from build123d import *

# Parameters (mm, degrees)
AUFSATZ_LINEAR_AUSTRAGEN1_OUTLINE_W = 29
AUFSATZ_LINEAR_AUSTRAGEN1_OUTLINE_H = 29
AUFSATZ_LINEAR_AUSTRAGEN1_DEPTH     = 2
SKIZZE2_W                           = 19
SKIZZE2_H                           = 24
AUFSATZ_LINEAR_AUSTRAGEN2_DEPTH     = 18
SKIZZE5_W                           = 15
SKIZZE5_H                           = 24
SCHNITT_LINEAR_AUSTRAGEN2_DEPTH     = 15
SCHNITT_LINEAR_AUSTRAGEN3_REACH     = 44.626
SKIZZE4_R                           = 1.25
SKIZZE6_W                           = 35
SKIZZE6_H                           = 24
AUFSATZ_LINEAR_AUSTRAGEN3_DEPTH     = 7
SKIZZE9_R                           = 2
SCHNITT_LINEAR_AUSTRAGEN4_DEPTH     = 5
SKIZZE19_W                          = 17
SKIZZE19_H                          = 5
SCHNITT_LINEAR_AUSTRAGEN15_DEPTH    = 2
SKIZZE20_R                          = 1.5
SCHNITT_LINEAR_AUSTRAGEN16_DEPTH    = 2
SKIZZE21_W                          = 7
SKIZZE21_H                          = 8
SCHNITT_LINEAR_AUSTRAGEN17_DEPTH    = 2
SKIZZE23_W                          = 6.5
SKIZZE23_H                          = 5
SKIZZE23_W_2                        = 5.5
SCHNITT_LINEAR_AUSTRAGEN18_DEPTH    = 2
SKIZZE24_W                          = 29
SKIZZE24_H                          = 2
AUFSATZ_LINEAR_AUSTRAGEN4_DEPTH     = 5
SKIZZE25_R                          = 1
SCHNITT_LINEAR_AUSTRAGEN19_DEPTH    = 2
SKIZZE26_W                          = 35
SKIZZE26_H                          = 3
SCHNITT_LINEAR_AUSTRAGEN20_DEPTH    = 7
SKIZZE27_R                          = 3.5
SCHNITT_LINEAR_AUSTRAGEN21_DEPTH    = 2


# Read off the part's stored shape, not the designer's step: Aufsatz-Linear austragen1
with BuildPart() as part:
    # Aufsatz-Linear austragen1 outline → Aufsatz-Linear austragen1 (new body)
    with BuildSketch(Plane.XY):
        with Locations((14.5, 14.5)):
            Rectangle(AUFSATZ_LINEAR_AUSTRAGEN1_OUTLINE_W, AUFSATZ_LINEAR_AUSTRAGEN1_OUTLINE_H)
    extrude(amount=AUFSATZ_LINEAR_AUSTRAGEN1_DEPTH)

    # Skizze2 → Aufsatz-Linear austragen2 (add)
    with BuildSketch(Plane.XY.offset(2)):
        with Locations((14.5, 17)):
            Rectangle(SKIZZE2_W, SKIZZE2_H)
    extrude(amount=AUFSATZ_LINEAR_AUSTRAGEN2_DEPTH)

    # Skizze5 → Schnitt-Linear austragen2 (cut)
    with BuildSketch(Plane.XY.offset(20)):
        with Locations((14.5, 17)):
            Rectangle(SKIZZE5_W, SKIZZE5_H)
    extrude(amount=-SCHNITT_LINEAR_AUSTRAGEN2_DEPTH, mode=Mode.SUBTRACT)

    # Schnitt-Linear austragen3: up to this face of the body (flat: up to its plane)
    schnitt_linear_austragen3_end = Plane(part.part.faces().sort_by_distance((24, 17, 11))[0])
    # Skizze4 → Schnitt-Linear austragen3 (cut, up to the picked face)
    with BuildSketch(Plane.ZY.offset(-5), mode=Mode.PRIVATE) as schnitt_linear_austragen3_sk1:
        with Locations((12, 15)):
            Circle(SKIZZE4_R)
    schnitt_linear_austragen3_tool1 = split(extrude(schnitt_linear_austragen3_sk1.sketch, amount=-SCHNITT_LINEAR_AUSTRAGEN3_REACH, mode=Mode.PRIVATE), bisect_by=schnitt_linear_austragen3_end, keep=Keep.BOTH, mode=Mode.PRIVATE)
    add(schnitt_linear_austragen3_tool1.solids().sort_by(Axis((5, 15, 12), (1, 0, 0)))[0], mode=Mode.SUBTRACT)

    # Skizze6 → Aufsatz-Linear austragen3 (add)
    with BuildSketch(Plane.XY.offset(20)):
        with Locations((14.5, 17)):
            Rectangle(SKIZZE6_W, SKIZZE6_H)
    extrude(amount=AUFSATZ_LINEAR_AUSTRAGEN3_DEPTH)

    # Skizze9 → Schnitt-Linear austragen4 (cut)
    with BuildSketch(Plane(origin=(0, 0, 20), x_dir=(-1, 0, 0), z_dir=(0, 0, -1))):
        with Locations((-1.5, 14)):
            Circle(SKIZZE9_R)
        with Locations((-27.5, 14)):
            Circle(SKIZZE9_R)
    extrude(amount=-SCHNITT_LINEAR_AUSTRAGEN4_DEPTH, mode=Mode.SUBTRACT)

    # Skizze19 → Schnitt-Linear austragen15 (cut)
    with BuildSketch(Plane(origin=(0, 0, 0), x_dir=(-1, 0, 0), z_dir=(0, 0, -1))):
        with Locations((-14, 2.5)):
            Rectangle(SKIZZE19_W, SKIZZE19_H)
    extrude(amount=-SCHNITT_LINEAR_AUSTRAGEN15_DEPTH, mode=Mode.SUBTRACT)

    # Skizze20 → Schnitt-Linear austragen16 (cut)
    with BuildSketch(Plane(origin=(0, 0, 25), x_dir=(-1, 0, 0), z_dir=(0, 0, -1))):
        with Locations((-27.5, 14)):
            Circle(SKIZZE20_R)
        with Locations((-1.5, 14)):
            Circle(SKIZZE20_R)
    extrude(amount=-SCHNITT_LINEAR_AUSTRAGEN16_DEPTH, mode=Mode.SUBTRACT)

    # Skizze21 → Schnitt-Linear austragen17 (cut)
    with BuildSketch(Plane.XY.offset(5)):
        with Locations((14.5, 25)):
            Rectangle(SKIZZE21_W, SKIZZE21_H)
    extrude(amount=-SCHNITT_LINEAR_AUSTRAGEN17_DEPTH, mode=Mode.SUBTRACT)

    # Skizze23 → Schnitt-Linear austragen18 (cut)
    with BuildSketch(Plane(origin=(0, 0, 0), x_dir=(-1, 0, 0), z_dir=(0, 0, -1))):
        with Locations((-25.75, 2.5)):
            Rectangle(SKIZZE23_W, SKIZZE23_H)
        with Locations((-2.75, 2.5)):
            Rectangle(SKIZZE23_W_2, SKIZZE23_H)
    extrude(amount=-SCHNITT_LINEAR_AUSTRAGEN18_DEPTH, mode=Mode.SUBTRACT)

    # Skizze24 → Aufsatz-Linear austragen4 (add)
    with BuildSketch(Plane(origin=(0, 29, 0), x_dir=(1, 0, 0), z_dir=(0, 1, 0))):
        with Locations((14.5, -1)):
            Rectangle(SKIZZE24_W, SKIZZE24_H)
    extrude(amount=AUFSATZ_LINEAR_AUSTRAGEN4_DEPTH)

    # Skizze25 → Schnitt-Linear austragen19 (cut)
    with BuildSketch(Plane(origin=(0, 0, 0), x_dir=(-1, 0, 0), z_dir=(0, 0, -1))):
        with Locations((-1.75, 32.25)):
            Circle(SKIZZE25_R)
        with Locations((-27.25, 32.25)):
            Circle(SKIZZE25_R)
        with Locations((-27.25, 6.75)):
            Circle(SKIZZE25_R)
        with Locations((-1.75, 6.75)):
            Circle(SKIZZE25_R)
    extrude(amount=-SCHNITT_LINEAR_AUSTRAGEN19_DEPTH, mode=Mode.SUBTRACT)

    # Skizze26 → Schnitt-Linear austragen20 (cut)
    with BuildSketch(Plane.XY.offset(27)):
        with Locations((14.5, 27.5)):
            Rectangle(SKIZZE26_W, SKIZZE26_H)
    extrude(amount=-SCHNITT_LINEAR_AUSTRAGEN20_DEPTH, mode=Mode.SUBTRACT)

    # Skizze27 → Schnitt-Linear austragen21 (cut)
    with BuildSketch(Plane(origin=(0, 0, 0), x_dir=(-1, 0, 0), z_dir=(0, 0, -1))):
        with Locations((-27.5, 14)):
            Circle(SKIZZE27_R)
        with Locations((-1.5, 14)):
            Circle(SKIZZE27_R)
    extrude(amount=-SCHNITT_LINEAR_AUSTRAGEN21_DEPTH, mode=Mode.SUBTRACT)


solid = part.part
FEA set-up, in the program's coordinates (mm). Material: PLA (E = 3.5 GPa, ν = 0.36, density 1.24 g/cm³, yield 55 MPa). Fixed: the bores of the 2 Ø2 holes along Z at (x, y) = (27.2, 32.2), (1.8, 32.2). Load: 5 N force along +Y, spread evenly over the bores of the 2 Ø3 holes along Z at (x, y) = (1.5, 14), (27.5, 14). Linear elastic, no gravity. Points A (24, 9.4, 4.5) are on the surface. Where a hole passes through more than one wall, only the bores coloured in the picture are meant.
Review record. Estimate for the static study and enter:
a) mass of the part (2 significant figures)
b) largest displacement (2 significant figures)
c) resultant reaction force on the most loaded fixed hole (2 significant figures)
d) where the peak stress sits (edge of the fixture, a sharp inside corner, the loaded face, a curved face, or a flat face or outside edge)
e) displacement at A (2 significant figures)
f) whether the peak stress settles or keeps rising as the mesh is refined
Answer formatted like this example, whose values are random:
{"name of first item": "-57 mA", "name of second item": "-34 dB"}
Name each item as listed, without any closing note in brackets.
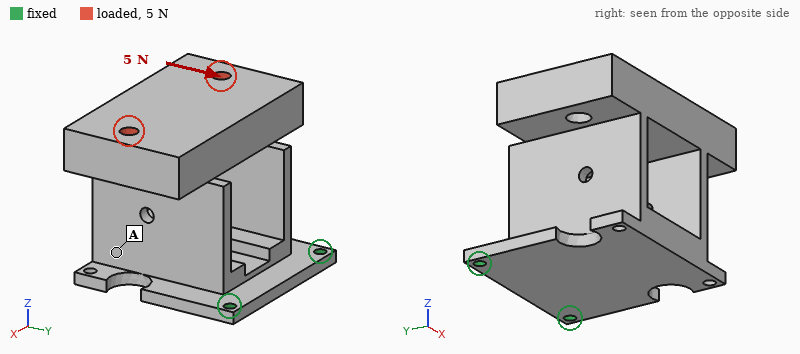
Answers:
{"mass of the part": "11 g", "largest displacement": "0.58 mm", "resultant reaction force on the most loaded fixed hole": "2.7 N", "where the peak stress sits": "edge of the fixture", "displacement at A": "0.33 mm", "whether the peak stress settles or keeps rising as the mesh is refined": "keeps rising"}
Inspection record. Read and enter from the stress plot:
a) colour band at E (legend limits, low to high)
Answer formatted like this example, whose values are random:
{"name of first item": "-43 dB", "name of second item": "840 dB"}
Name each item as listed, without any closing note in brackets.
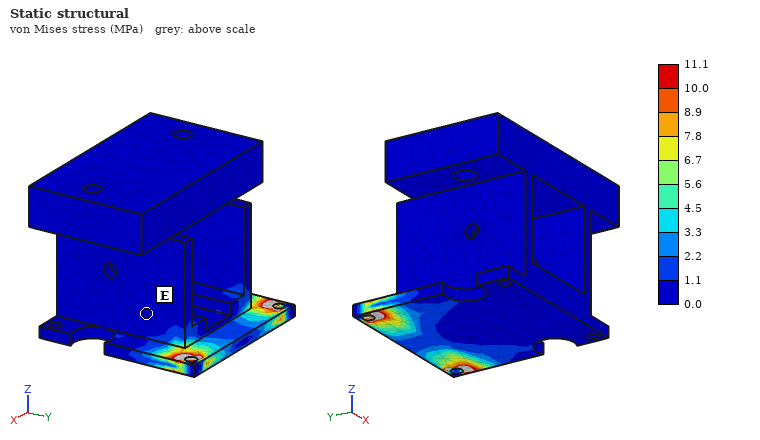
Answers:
{"colour band at E": "0.0 to 1.1 MPa"}
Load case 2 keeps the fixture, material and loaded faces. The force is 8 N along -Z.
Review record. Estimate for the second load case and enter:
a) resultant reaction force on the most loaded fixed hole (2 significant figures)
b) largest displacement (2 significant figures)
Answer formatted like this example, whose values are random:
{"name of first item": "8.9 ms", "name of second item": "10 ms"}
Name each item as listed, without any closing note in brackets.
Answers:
{"resultant reaction force on the most loaded fixed hole": "4.0 N", "largest displacement": "0.60 mm"}
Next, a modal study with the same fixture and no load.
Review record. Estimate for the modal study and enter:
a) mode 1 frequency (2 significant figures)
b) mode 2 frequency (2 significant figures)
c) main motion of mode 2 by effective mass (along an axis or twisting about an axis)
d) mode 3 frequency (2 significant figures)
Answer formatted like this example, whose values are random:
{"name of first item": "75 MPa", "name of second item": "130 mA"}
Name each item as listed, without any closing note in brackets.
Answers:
{"mode 1 frequency": "180 Hz", "mode 2 frequency": "640 Hz", "main motion of mode 2 by effective mass": "along X", "mode 3 frequency": "1700 Hz"}
